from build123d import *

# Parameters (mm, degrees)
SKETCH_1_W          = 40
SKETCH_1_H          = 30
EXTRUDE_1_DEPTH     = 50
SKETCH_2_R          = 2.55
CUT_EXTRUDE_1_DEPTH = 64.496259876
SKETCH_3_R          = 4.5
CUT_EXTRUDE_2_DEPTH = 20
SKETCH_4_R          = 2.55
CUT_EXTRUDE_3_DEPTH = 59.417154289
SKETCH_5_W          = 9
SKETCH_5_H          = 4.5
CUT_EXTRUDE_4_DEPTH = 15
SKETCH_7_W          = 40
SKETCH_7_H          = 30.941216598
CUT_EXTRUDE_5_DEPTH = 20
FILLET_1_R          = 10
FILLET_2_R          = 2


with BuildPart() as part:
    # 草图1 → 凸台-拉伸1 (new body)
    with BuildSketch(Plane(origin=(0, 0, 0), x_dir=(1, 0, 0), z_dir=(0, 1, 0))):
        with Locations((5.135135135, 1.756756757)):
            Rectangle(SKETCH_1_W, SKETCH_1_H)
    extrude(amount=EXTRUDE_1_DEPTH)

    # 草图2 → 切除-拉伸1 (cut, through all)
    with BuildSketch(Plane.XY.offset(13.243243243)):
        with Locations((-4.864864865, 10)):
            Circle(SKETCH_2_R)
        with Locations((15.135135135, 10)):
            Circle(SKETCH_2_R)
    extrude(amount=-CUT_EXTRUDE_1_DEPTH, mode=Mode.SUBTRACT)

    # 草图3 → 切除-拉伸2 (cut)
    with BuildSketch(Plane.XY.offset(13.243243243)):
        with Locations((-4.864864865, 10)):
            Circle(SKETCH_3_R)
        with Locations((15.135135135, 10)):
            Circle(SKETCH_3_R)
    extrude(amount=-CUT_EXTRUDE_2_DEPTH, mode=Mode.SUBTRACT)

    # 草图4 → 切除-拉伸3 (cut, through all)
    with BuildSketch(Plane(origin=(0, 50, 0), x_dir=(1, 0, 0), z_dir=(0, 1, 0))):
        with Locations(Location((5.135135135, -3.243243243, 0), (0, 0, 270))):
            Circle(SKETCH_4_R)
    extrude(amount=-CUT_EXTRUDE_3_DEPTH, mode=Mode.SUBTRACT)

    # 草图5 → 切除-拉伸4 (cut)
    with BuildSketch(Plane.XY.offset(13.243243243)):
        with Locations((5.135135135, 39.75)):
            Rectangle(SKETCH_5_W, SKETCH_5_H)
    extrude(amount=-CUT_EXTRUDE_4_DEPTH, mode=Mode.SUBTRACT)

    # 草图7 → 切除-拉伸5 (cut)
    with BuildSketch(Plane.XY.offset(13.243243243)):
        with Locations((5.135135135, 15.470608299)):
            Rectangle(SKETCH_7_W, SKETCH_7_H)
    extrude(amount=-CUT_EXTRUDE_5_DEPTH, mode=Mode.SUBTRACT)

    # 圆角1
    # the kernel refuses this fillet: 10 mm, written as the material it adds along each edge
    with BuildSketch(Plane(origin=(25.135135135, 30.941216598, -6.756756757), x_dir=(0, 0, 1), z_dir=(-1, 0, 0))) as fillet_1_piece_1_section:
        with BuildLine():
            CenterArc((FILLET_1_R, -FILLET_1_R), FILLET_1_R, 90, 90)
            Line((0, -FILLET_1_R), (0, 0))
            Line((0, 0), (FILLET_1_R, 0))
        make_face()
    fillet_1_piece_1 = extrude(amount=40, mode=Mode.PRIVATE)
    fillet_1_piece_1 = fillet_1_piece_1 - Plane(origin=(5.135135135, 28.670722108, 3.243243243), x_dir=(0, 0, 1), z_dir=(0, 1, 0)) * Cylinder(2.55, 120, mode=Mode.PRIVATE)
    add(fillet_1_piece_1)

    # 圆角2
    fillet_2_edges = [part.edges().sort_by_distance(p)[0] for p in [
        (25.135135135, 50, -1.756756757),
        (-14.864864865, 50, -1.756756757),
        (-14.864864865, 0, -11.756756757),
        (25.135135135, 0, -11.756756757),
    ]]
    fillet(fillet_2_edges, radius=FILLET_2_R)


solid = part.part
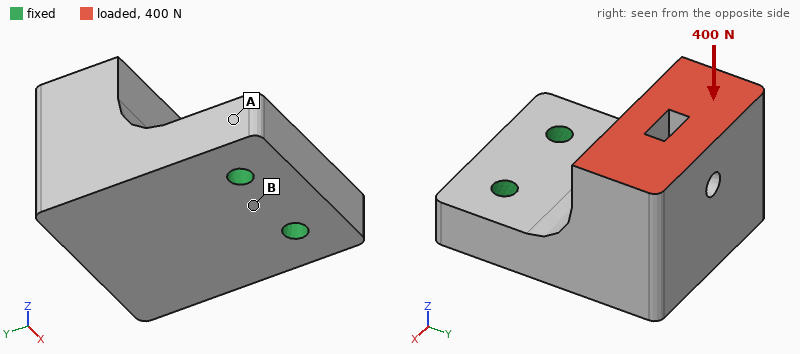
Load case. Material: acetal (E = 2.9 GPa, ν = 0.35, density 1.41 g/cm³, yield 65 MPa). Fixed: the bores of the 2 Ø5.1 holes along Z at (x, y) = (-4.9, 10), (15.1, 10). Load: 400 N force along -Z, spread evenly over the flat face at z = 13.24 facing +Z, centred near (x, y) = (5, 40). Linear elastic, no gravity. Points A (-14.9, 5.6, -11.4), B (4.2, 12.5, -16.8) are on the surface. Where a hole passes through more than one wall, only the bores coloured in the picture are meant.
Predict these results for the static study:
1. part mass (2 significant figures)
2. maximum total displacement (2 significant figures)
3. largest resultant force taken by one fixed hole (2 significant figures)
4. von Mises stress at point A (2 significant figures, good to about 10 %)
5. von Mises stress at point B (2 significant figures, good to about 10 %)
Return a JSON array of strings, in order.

["49 g", "0.70 mm", "200 N", "3.0 MPa", "8.7 MPa"]
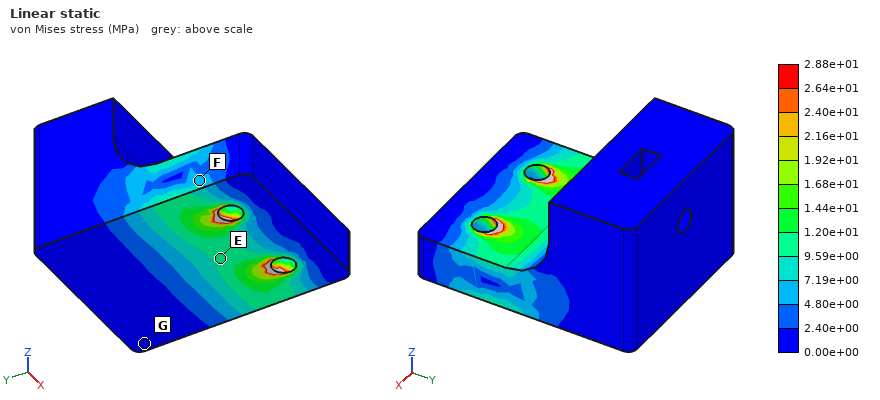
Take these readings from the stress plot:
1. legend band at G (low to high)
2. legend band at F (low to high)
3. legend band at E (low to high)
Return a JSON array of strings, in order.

["0.00e+00 to 2.40e+00 MPa", "4.80e+00 to 7.19e+00 MPa", "9.59e+00 to 1.20e+01 MPa"]
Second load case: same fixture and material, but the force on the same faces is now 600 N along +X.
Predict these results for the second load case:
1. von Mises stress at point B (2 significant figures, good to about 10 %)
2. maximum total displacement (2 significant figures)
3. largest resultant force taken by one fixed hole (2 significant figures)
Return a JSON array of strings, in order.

["3.9 MPa", "0.48 mm", "970 N"]
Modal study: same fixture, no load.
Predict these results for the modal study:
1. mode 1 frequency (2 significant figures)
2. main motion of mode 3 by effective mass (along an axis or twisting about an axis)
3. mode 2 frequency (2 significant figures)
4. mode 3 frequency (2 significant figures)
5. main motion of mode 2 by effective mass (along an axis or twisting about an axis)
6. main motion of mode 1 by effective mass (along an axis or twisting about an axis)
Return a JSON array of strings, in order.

["760 Hz", "along X", "1600 Hz", "2400 Hz", "along X", "along Z"]
